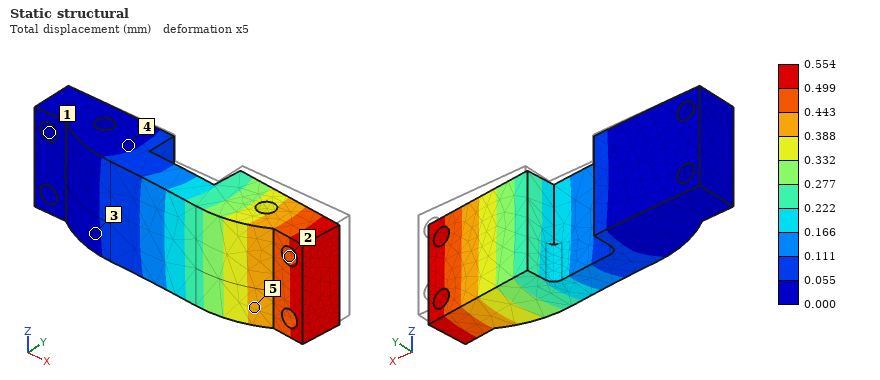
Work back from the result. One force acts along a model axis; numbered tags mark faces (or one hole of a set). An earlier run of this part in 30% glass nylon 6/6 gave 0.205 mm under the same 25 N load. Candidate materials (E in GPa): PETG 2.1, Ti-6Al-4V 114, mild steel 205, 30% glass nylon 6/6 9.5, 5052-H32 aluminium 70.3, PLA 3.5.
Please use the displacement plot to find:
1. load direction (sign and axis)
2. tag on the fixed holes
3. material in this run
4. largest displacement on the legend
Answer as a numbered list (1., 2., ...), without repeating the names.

1. -Y
2. 1
3. PLA
4. 0.554 mm
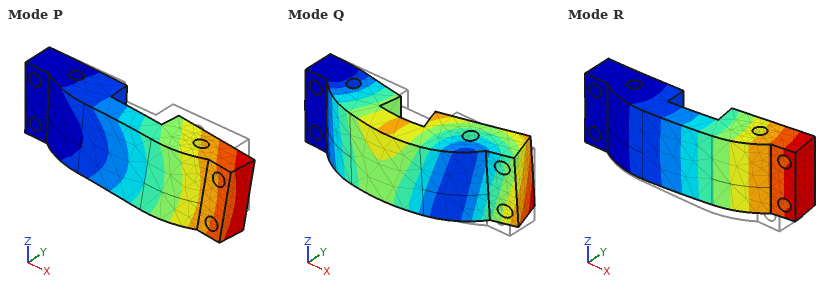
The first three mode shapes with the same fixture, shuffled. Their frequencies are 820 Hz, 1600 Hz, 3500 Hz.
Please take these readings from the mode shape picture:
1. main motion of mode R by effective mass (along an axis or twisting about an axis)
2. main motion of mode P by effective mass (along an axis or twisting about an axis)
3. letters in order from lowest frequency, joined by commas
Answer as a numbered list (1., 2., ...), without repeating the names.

1. along Y
2. along Z
3. R, P, Q
